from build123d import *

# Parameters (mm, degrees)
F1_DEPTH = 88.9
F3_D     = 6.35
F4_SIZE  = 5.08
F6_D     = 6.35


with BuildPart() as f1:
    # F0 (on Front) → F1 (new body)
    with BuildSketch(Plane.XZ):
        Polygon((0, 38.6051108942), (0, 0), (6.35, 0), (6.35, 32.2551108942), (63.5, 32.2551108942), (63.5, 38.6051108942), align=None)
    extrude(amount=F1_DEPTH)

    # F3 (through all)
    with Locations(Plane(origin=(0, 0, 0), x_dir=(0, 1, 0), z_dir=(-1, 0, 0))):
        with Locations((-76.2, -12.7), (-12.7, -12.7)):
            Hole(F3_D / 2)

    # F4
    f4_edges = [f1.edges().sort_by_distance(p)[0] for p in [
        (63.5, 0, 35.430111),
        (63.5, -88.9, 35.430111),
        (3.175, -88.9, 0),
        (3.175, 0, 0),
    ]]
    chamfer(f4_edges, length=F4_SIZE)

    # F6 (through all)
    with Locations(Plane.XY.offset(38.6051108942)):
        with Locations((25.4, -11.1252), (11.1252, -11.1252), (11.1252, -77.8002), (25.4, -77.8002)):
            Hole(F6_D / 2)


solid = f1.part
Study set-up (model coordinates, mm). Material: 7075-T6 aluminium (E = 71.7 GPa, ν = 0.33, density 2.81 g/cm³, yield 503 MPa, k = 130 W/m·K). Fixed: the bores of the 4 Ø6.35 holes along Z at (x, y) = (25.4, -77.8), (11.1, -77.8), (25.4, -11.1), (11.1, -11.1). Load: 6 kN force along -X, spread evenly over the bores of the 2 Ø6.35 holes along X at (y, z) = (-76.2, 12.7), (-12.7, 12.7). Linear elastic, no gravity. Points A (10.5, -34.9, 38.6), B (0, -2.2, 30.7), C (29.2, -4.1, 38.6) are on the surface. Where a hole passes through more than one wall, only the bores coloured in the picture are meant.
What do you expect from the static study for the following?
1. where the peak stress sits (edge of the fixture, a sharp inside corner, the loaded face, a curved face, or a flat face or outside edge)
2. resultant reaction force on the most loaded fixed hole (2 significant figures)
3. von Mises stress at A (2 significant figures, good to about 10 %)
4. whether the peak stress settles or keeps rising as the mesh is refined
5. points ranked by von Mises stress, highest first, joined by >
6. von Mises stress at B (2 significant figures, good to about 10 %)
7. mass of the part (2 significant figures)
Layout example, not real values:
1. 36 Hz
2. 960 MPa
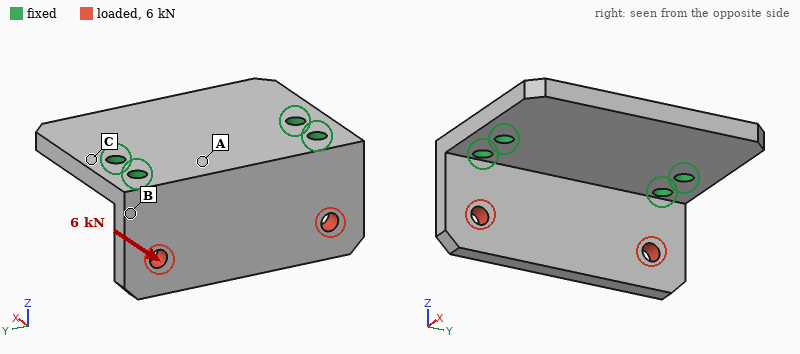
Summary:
1. edge of the fixture
2. 2.9 kN
3. 100 MPa
4. keeps rising
5. B > A > C
6. 190 MPa
7. 150 g
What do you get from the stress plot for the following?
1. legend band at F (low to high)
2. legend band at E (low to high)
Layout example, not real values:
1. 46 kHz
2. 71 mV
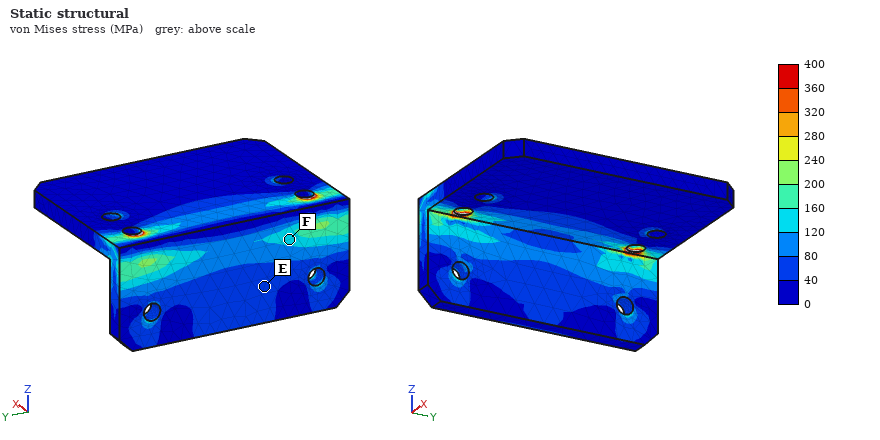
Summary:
1. 120 to 160 MPa
2. 40 to 80 MPa
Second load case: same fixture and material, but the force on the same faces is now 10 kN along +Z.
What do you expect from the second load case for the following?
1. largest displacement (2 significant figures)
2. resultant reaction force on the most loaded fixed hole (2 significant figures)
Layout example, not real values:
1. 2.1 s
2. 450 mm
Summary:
1. 0.12 mm
2. 5.5 kN
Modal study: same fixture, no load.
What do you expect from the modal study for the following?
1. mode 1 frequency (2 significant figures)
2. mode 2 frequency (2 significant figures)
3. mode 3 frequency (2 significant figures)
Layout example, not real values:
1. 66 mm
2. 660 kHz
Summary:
1. 3000 Hz
2. 3200 Hz
3. 4900 Hz
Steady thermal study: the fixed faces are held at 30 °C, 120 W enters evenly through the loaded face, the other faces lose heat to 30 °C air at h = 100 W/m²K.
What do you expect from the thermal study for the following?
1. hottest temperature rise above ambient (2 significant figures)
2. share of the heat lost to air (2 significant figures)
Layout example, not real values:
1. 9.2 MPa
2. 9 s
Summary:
1. 63 K
2. 25 %
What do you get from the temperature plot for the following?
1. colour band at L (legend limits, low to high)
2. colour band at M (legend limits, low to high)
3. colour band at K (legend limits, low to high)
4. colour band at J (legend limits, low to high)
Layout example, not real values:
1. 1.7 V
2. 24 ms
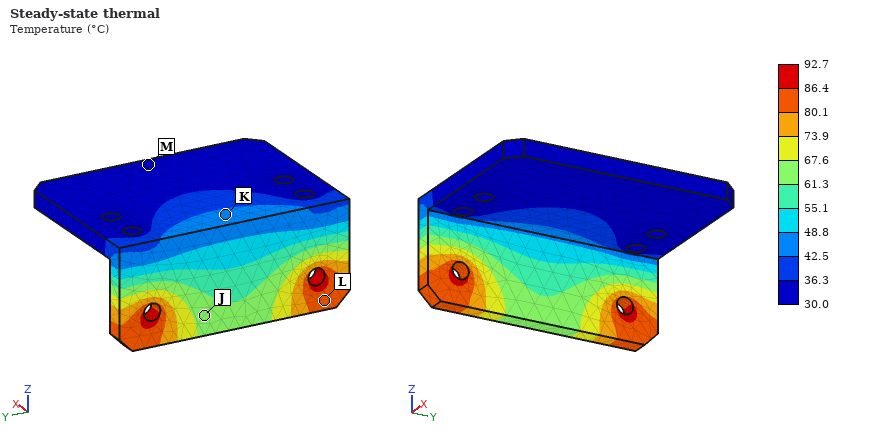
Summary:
1. 80.1 to 86.4 °C
2. 30.0 to 36.3 °C
3. 42.5 to 48.8 °C
4. 61.3 to 67.6 °C
